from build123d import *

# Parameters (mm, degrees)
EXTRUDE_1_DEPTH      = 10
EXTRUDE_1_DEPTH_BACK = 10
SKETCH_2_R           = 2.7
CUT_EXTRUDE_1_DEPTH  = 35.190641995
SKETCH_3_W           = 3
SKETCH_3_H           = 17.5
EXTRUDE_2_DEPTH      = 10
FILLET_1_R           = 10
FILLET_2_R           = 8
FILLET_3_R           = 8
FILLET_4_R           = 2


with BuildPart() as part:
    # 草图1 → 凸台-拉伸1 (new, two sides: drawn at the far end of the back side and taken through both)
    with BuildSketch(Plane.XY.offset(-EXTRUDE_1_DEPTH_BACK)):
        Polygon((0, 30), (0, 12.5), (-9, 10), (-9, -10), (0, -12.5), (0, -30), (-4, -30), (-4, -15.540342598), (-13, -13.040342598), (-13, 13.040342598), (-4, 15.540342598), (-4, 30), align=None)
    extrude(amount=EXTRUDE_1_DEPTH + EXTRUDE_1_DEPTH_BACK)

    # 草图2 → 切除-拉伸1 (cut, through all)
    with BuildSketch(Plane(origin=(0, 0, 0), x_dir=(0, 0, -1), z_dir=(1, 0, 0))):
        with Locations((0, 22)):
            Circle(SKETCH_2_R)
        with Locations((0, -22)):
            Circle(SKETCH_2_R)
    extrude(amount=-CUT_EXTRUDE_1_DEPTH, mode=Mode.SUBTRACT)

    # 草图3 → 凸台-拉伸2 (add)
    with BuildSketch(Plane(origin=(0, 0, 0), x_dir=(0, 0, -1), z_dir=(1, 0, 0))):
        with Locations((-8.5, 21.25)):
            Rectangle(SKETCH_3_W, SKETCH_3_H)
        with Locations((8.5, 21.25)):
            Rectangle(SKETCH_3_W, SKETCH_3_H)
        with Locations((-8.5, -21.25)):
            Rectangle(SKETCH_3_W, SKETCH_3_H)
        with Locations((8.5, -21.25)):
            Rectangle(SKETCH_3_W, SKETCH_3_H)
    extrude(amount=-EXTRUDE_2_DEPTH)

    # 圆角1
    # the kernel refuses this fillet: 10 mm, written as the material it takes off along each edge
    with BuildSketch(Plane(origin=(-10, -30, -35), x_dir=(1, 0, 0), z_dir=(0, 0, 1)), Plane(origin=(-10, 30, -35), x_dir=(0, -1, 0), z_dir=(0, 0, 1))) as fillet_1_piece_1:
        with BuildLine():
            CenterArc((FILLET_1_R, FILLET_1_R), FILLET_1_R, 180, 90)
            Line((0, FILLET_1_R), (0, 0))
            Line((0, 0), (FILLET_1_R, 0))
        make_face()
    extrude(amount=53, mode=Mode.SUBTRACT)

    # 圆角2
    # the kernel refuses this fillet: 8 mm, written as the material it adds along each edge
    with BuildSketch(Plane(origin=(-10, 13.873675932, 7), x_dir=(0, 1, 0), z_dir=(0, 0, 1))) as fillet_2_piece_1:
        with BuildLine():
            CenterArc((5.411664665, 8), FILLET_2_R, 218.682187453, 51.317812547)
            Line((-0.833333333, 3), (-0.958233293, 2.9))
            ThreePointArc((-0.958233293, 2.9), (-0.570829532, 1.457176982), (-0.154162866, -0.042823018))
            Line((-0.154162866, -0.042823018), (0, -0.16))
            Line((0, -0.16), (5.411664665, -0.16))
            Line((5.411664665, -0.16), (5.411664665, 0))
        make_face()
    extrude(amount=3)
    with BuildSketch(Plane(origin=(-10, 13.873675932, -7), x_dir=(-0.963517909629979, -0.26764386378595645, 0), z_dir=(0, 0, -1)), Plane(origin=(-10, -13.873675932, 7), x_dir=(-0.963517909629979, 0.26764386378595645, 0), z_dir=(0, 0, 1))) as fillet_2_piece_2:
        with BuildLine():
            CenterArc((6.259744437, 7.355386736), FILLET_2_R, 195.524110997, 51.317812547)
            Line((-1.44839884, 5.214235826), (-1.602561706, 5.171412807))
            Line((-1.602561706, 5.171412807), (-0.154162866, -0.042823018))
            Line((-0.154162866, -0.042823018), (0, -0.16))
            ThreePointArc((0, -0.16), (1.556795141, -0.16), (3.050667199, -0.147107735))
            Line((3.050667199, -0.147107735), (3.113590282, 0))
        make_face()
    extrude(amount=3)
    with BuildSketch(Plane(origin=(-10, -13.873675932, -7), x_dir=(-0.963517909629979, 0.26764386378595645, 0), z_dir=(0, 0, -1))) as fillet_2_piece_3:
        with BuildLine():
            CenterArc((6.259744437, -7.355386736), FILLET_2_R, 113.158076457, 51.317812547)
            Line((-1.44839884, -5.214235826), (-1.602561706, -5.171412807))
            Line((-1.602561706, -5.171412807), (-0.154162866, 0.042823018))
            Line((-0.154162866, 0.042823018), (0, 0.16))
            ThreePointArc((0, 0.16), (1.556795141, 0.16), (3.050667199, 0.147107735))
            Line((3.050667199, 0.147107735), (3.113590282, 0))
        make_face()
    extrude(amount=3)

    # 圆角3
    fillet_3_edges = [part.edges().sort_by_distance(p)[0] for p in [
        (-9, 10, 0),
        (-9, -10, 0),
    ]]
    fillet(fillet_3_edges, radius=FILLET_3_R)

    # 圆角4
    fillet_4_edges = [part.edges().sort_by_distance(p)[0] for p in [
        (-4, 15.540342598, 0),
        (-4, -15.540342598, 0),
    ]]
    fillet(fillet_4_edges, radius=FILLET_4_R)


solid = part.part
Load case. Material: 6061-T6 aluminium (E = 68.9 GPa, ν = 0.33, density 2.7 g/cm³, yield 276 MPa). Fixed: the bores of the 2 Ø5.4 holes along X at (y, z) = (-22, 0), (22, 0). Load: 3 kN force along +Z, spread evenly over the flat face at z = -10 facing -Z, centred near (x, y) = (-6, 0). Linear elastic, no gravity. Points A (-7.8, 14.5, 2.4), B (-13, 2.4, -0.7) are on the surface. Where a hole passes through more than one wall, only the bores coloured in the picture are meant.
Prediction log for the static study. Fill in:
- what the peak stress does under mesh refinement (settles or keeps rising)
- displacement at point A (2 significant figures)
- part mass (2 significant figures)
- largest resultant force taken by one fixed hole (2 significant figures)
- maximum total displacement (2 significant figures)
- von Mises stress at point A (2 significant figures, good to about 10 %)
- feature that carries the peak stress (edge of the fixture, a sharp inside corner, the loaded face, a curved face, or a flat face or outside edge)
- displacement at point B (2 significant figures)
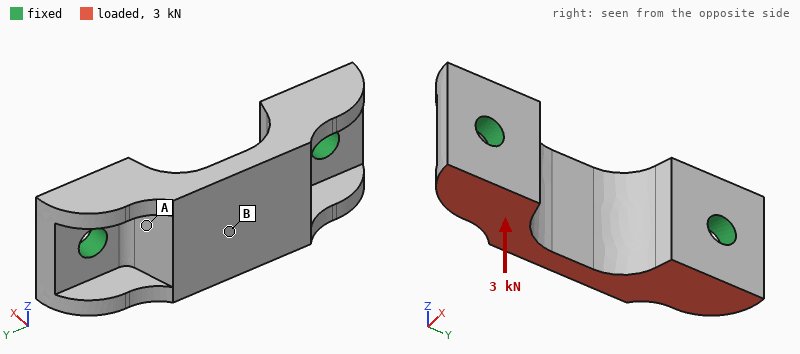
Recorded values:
keeps rising
22 µm
19 g
1.5 kN
48 µm
32 MPa
edge of the fixture
38 µm
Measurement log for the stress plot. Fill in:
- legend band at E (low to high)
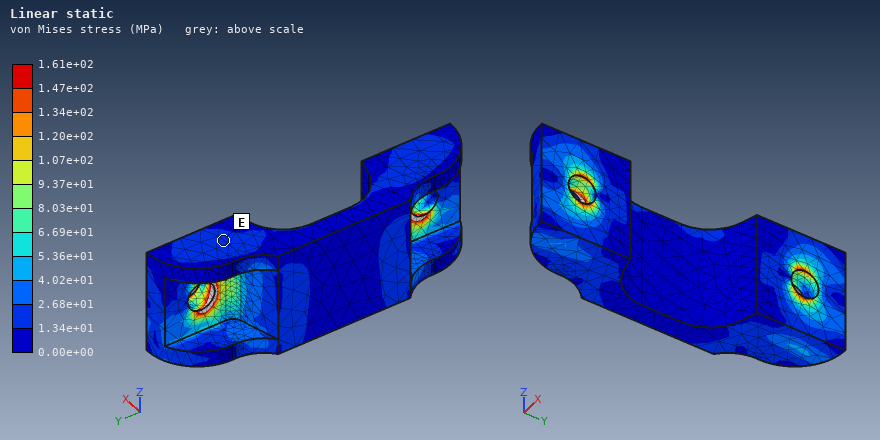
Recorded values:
1.34e+01 to 2.68e+01 MPa
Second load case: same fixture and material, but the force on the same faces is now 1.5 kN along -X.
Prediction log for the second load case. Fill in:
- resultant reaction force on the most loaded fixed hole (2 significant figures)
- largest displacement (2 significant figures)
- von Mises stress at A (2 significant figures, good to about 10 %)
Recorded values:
800 N
41 µm
17 MPa
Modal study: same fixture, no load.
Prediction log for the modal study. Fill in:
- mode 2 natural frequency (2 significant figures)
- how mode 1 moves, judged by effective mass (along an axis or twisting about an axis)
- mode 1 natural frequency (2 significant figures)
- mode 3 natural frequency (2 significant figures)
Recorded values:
19 kHz
along Z
10 kHz
20 kHz
